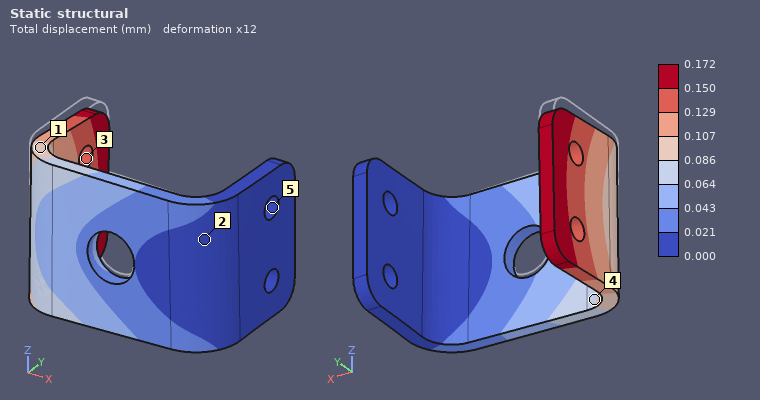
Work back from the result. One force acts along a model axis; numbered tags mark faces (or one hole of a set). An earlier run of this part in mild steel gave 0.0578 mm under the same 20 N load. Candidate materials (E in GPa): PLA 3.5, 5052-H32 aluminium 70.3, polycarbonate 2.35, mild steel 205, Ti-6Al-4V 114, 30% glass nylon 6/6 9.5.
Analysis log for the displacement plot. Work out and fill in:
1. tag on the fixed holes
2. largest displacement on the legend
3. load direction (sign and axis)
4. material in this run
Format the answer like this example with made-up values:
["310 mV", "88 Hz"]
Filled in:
["5", "0.172 mm", "-Z", "5052-H32 aluminium"]
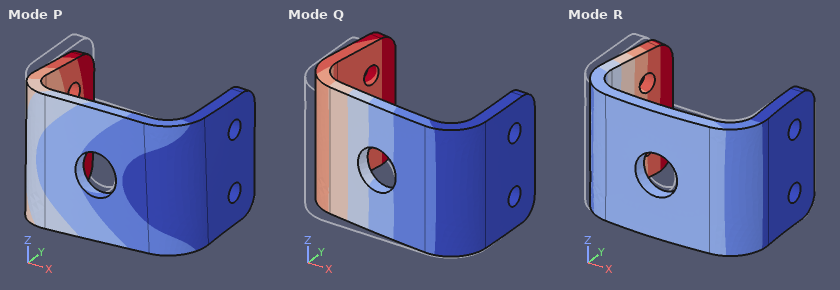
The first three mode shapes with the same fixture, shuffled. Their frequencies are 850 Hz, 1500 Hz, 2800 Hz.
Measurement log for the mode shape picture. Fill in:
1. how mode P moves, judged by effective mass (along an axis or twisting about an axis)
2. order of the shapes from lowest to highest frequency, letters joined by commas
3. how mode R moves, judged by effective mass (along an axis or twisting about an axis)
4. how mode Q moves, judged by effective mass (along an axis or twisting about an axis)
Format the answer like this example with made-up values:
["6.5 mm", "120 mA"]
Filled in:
["along Z", "Q, P, R", "along X", "along Y"]
